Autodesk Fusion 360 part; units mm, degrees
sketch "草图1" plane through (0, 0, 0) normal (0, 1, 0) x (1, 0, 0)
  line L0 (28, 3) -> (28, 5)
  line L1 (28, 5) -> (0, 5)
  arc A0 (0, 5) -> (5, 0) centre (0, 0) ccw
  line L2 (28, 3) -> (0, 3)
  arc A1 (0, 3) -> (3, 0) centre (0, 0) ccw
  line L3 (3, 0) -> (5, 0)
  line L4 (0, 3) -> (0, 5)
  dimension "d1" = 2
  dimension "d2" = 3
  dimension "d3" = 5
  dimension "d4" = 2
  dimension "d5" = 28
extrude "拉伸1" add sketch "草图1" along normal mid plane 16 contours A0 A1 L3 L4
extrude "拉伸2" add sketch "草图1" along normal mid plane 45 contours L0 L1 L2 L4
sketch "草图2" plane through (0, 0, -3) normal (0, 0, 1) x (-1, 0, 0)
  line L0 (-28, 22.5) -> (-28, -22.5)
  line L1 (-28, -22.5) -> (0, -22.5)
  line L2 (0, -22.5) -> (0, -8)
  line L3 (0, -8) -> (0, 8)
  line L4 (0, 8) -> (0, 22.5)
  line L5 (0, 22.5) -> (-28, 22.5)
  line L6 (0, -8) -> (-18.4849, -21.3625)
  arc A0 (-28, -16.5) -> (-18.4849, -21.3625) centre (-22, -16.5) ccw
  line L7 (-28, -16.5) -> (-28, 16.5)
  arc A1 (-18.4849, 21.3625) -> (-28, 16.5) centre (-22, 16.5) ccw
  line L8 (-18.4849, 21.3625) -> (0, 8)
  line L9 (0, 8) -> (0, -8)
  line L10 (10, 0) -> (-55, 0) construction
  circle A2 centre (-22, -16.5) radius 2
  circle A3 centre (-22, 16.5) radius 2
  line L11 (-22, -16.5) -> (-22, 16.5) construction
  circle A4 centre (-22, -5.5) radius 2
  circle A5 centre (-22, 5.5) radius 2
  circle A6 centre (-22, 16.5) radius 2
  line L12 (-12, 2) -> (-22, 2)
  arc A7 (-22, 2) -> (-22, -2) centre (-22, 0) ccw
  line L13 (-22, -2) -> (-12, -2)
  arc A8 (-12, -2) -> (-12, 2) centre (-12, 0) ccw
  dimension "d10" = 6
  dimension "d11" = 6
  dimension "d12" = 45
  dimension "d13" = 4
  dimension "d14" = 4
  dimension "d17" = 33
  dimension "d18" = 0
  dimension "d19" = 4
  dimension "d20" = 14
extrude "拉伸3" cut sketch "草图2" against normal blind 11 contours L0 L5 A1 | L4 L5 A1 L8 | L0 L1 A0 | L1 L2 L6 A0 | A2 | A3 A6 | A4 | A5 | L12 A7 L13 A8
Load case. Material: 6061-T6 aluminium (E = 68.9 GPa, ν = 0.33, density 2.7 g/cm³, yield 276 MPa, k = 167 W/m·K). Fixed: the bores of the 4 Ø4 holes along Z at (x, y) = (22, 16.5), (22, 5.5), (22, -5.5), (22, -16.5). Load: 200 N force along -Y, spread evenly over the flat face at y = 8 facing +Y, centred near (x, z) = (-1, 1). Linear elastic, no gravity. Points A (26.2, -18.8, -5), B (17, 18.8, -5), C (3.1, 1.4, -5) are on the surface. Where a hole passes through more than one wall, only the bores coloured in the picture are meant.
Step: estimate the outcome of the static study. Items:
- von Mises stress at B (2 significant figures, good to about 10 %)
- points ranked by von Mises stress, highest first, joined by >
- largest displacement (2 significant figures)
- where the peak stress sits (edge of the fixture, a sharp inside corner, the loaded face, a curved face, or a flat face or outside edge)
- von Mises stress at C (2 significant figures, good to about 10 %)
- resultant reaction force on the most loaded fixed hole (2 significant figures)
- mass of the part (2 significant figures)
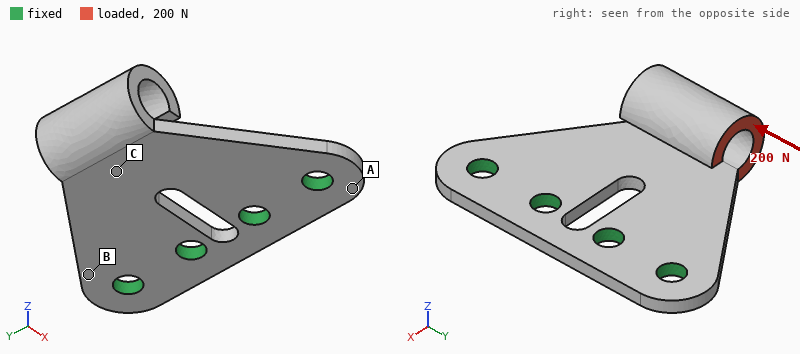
34 MPa
C > B > A
0.14 mm
a curved face
45 MPa
140 N
6.2 g
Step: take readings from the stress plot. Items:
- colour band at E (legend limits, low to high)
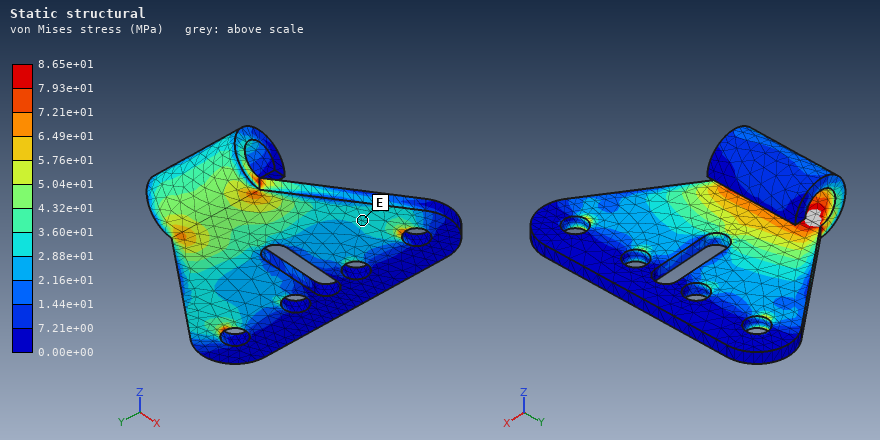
2.88e+01 to 3.60e+01 MPa
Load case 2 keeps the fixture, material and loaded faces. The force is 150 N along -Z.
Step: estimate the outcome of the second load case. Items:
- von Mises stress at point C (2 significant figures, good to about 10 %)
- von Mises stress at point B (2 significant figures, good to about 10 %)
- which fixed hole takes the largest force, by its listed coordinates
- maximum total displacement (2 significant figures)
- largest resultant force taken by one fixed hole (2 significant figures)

79 MPa
120 MPa
(22, 5.5)
0.60 mm
66 N
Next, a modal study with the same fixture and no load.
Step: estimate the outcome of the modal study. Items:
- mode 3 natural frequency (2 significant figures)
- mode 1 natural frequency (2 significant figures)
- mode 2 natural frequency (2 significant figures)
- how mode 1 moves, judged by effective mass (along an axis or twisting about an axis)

5800 Hz
2000 Hz
4700 Hz
along Z
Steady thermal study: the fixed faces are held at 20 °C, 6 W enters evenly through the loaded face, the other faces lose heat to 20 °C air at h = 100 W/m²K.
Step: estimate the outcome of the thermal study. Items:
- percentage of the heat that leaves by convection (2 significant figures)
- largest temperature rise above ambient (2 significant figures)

29 %
25 K
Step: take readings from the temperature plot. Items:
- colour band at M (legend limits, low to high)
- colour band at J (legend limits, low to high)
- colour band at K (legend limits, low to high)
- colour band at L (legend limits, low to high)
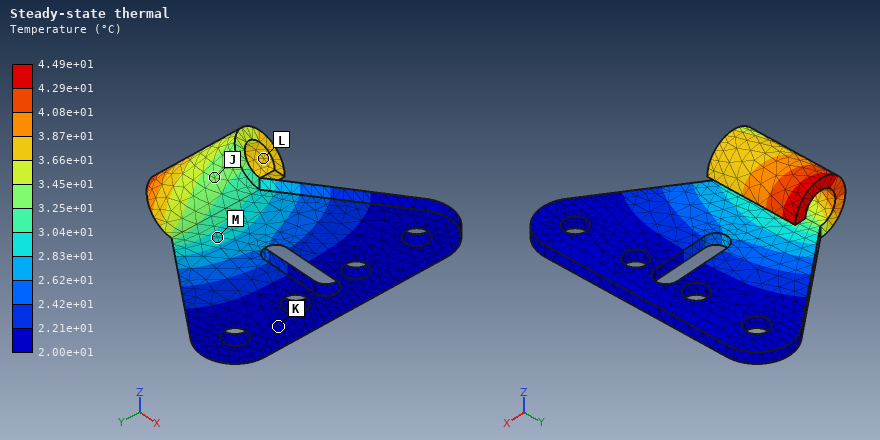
2.83e+01 to 3.04e+01 °C
3.25e+01 to 3.45e+01 °C
2.00e+01 to 2.21e+01 °C
3.66e+01 to 3.87e+01 °C
